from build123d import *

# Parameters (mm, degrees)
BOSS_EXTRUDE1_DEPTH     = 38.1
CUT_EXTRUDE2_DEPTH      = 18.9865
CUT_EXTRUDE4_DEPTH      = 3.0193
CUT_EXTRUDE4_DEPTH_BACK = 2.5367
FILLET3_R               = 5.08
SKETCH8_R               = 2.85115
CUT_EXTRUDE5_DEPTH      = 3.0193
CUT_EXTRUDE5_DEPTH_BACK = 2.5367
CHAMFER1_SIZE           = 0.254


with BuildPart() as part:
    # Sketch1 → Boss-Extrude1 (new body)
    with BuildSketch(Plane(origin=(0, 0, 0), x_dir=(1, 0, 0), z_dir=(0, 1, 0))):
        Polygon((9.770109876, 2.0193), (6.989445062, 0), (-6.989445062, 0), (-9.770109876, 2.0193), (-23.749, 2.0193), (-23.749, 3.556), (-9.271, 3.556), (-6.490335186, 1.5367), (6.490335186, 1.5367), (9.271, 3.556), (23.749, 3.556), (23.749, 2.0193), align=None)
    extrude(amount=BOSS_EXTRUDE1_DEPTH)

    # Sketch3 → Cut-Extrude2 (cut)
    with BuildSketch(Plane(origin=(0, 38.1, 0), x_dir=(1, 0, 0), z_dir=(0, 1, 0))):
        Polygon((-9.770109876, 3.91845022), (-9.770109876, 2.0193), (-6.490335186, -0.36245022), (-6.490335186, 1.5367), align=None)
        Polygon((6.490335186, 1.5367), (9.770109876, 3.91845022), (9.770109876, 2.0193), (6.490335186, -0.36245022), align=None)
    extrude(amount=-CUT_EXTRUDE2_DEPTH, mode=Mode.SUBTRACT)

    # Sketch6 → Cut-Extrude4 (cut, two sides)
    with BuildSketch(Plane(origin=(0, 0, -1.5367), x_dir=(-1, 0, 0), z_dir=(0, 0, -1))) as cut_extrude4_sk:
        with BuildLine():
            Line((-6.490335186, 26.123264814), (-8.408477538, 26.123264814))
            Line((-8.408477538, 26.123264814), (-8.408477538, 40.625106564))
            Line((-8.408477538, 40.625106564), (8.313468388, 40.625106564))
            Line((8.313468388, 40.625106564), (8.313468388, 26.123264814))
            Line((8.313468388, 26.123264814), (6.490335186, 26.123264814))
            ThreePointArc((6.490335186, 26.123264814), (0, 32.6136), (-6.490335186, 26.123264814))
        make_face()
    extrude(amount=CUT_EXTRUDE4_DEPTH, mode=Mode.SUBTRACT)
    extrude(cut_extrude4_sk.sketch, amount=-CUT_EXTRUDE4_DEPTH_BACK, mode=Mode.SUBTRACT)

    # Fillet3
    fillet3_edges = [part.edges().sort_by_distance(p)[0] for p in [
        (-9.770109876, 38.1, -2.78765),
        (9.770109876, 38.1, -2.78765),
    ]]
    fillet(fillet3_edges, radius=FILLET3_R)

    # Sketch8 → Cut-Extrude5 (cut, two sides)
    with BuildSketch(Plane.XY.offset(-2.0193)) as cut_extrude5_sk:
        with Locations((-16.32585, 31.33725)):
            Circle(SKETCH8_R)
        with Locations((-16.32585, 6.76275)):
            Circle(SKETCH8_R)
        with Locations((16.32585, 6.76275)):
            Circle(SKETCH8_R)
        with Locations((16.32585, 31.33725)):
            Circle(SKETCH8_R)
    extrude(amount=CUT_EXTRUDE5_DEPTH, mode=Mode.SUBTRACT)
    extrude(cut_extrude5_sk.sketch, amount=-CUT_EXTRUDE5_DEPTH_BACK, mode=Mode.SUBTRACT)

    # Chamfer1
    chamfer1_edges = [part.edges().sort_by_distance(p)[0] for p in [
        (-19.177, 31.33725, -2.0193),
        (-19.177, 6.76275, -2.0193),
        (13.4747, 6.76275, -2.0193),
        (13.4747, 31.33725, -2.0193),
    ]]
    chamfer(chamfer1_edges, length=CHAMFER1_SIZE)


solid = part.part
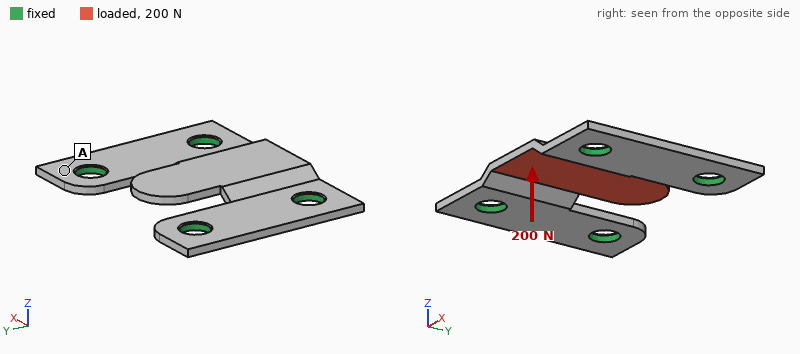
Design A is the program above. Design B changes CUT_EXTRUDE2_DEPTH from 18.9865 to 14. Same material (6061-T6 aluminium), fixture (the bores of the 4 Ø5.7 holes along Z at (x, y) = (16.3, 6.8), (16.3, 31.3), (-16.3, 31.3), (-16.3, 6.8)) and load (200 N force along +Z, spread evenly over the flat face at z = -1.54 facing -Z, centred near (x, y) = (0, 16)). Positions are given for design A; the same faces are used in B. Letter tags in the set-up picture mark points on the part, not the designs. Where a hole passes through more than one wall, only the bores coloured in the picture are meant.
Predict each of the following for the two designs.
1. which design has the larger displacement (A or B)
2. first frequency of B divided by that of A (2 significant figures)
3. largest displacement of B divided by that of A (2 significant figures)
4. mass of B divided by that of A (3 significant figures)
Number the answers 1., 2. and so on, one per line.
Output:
1. A
2. 1.8
3. 0.30
4. 1.03
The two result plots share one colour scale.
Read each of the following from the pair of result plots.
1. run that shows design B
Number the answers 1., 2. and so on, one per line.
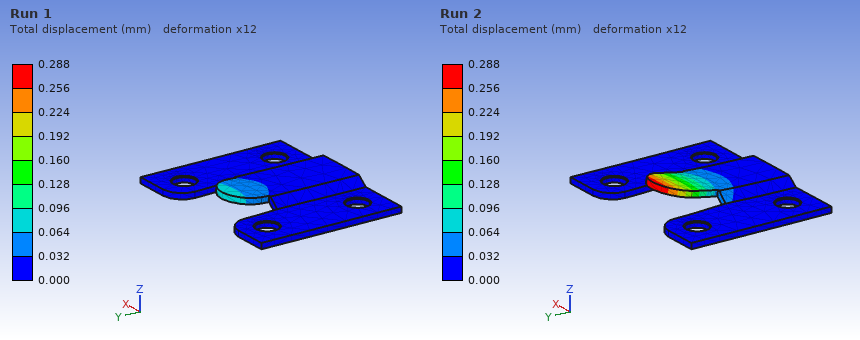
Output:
1. Run 1
